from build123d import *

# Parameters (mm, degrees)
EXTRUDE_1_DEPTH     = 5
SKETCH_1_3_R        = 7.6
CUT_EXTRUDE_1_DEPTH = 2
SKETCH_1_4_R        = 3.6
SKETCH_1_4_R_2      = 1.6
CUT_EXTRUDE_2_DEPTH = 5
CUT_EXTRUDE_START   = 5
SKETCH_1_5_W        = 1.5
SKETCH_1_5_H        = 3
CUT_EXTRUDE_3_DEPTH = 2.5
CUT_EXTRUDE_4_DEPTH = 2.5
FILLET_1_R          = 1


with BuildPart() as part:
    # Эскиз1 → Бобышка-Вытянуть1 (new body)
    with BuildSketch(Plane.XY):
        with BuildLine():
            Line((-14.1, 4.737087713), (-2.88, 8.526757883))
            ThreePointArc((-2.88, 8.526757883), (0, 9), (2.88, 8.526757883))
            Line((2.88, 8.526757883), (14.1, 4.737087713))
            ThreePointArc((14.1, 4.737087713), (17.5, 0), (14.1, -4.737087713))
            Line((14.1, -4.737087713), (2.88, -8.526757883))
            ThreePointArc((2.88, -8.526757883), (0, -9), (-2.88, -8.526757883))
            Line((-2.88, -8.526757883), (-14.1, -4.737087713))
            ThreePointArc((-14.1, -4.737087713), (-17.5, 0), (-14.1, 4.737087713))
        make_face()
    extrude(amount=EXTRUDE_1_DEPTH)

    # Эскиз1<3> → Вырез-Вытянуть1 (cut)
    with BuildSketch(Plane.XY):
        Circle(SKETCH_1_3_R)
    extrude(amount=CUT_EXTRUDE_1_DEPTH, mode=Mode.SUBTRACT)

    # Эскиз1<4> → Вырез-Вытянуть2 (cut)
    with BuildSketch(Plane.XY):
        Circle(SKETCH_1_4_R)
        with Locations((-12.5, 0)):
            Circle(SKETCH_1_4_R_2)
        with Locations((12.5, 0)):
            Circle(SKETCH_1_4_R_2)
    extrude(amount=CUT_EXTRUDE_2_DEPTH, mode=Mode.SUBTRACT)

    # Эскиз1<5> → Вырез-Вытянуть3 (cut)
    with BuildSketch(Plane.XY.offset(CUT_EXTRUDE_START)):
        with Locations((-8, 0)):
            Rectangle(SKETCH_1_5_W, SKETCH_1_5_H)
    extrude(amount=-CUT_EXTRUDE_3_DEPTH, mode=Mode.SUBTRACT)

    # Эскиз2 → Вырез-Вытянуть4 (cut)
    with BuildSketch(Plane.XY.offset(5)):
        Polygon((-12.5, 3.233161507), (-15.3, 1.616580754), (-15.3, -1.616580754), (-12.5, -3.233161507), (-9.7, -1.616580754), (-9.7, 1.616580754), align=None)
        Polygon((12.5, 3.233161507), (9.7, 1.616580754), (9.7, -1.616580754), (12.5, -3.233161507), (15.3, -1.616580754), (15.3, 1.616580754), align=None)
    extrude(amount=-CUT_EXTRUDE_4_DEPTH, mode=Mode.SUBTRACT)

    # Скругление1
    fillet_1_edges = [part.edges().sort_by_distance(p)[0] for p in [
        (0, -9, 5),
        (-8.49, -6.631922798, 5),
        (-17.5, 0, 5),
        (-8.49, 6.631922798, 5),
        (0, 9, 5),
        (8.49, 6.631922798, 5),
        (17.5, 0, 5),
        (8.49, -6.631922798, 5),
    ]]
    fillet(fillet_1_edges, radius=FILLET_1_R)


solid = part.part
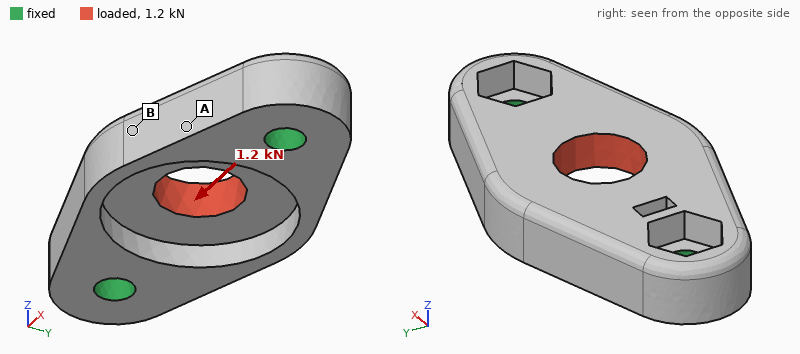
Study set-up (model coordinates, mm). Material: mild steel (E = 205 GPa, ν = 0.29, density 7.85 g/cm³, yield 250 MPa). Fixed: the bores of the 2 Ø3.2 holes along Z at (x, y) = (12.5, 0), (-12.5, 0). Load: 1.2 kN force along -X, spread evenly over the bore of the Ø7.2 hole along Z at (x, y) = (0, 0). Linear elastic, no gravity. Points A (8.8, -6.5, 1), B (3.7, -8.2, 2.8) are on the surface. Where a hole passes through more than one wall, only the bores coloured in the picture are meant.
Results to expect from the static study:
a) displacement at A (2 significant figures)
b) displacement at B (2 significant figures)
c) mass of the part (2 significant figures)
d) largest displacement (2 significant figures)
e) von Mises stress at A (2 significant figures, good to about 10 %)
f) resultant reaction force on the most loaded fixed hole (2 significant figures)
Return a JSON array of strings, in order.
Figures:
["0.73 µm", "1.0 µm", "12 g", "1.6 µm", "11 MPa", "610 N"]
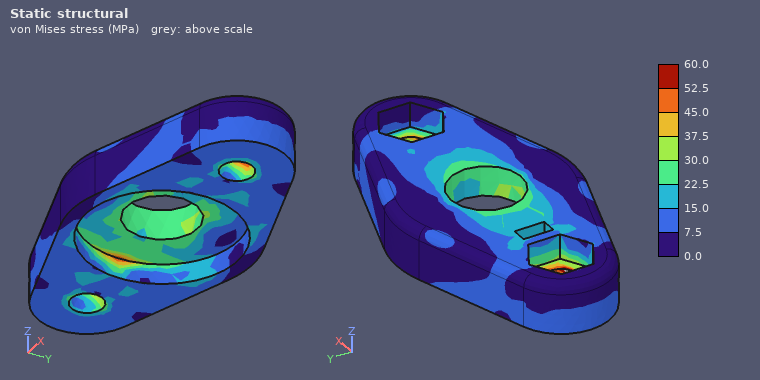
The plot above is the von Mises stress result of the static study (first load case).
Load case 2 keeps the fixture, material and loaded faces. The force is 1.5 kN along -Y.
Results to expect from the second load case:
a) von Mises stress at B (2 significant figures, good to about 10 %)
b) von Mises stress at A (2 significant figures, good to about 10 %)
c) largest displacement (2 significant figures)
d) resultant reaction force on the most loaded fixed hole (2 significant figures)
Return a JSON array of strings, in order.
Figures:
["41 MPa", "25 MPa", "9.6 µm", "760 N"]
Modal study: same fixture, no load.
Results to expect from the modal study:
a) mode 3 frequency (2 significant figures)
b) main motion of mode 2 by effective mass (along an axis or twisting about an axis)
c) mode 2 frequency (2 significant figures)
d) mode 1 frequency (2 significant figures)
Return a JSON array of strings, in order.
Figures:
["46 kHz", "along Z", "25 kHz", "20 kHz"]
